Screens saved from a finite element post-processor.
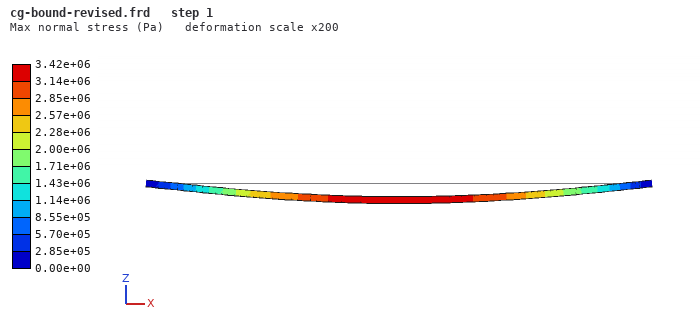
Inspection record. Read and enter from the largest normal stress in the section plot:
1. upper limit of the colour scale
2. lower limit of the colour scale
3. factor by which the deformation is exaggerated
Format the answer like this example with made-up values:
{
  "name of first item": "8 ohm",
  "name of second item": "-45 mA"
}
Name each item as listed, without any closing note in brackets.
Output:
{
  "upper limit of the colour scale": "3.42e+06 Pa",
  "lower limit of the colour scale": "0.00e+00 Pa",
  "factor by which the deformation is exaggerated": "200"
}
